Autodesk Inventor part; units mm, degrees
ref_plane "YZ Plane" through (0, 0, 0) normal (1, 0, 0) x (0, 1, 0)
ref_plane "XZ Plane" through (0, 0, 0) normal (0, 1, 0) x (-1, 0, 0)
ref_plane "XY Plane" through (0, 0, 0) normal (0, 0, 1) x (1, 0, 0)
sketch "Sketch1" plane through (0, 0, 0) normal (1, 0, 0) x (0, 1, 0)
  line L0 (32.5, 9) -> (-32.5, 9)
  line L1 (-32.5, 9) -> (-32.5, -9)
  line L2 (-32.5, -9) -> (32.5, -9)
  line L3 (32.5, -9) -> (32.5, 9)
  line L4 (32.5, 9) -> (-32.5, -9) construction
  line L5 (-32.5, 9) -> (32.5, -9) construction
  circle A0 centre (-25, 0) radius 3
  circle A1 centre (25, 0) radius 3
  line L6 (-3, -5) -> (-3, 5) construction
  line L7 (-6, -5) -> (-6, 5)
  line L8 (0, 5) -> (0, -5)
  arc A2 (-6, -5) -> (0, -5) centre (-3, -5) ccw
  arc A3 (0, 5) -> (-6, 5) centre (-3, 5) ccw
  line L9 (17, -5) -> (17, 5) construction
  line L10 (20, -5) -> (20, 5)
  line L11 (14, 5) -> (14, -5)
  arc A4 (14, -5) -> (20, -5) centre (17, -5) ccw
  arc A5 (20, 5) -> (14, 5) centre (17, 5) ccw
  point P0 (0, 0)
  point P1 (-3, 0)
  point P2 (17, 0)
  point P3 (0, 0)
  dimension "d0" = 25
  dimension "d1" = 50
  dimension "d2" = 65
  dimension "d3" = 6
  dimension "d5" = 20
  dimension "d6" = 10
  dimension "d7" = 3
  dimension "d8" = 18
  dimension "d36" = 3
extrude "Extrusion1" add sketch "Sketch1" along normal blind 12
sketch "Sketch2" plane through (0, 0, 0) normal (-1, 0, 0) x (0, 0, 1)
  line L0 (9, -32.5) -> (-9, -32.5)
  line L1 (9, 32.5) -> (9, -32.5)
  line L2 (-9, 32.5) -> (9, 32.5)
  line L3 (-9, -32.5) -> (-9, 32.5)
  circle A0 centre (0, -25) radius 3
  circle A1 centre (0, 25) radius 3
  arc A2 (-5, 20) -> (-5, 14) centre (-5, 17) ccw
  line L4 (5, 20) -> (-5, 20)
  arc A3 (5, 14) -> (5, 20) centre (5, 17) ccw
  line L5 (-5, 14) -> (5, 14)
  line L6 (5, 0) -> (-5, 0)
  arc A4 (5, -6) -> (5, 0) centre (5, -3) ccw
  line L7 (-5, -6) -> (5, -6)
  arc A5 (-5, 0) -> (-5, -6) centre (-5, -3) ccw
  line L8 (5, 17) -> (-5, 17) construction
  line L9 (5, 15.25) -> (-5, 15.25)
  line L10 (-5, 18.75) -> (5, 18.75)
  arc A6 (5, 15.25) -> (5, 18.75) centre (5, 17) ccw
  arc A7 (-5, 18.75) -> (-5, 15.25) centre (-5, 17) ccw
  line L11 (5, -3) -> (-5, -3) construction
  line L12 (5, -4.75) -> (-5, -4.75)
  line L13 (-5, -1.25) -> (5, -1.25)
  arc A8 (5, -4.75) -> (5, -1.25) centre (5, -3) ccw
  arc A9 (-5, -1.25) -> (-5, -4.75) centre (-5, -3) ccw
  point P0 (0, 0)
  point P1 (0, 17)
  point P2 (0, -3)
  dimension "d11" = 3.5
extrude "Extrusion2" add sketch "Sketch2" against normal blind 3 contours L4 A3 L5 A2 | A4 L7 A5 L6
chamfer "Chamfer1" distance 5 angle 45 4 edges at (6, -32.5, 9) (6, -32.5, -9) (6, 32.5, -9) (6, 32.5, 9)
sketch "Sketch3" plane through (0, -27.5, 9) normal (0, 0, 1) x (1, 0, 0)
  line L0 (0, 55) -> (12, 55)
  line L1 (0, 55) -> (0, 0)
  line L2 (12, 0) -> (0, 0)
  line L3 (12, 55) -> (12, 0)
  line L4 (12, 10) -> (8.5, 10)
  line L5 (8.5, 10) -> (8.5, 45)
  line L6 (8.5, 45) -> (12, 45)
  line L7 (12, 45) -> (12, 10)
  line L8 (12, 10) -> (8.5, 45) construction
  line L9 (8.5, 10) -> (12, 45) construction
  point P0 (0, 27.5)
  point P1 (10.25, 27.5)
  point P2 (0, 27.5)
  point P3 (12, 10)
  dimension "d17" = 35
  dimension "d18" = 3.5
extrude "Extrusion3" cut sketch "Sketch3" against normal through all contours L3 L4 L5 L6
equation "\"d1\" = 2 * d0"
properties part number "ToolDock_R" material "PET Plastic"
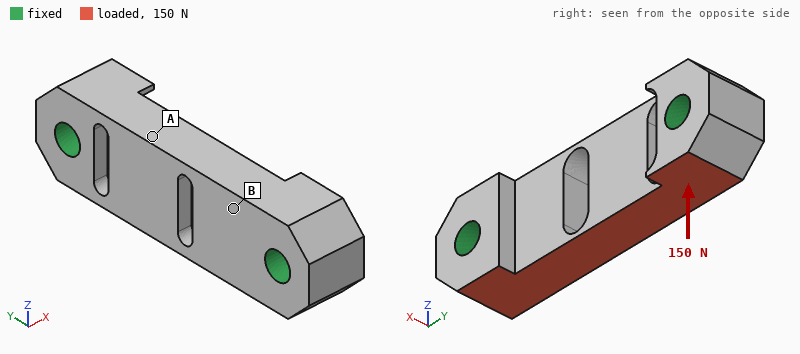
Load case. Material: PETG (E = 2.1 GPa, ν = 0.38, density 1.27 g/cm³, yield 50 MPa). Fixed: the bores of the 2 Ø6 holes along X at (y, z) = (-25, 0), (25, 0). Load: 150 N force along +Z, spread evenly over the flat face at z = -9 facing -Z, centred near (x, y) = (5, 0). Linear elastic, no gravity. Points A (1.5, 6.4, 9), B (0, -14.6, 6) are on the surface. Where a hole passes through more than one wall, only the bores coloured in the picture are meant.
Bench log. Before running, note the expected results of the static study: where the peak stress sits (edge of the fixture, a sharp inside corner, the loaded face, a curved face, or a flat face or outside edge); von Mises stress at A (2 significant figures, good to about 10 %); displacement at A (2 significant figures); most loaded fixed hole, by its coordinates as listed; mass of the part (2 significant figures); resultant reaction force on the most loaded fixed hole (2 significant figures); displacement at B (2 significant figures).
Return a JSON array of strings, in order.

["a curved face", "1.2 MPa", "37 µm", "(-25, 0)", "12 g", "83 N", "11 µm"]
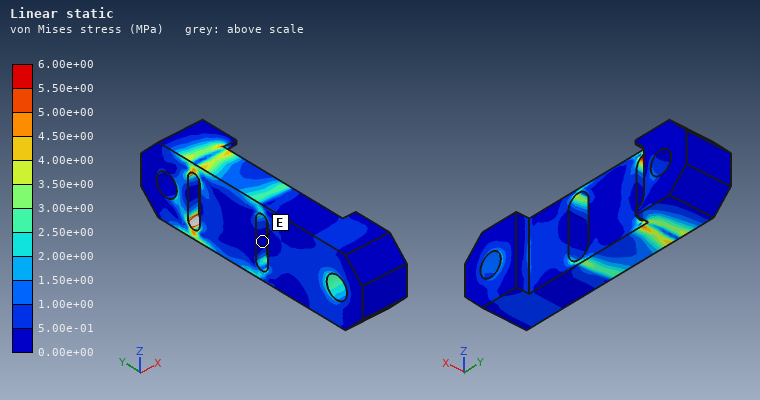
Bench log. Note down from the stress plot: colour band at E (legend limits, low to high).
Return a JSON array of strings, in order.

["0.00e+00 to 5.00e-01 MPa"]
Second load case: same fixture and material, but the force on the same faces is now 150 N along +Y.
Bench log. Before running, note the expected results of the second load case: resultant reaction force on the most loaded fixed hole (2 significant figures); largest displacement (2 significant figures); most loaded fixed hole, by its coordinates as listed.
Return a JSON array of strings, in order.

["90 N", "15 µm", "(-25, 0)"]
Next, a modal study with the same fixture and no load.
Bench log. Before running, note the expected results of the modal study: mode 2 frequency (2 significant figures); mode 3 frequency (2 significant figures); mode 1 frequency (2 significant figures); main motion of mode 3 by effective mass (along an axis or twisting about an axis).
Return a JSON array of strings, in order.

["3500 Hz", "5800 Hz", "3400 Hz", "twisting about Y"]
